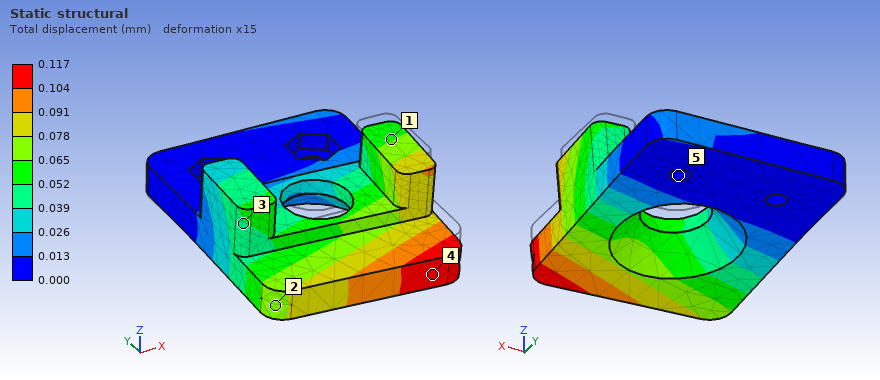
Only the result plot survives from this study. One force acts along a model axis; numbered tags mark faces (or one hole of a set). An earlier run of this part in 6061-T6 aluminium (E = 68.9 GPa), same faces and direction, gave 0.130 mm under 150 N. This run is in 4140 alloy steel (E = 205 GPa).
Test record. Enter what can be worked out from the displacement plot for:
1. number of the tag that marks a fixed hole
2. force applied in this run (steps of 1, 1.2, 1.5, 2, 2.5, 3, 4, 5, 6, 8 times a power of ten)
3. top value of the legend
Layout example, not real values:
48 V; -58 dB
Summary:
5; 400 N; 0.117 mm
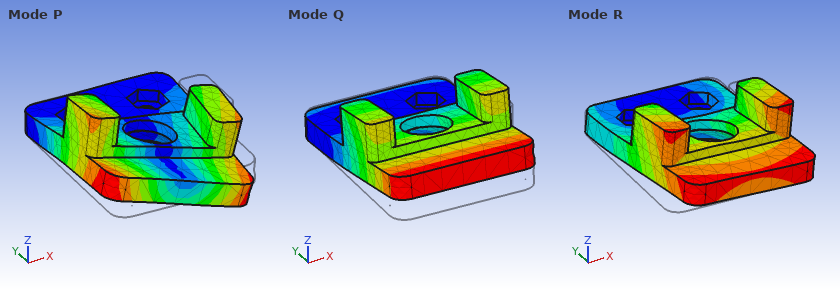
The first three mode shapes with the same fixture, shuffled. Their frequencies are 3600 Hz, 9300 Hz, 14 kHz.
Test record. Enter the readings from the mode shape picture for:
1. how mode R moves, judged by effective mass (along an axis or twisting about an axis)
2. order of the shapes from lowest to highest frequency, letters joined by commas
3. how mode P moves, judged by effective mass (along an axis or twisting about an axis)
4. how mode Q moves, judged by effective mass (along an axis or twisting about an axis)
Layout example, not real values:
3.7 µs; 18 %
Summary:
along X; Q, P, R; twisting about Y; along Z
